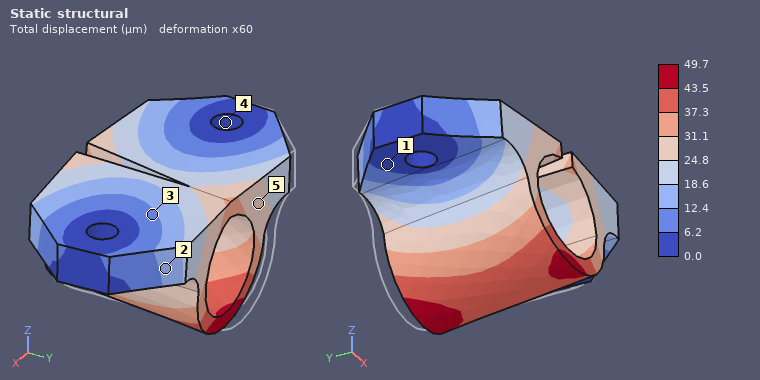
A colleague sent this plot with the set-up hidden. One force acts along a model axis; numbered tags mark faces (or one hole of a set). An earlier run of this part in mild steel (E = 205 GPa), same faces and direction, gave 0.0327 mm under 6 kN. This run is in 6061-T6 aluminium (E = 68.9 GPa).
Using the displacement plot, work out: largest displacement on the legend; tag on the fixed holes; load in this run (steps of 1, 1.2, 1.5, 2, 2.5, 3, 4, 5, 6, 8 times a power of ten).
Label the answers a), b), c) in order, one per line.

a) 49.7 µm
b) 4
c) 3 kN
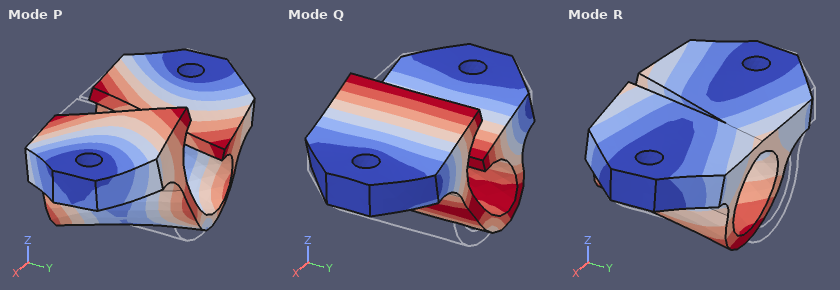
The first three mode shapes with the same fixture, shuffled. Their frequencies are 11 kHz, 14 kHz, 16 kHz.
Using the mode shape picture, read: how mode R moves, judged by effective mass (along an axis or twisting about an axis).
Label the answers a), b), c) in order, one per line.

a) along Y
